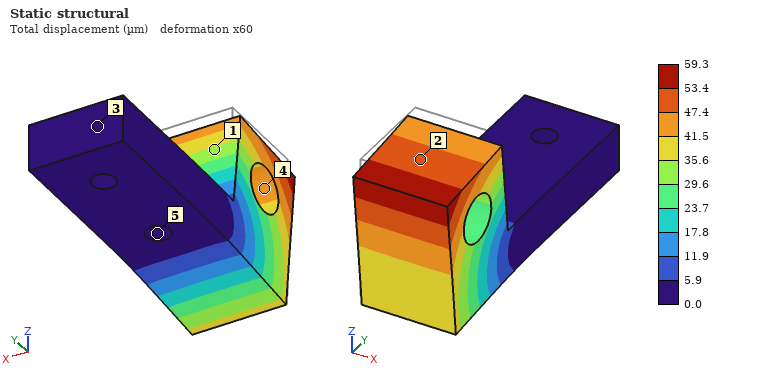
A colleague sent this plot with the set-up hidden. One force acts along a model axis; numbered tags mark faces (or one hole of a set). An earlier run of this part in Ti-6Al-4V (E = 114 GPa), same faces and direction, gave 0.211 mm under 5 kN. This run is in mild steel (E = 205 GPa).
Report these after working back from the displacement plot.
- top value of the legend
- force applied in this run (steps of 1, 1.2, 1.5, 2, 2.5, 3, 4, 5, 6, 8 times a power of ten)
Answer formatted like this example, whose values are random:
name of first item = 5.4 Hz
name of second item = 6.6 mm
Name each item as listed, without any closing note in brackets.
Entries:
top value of the legend = 59.3 µm
force applied in this run = 2.5 kN
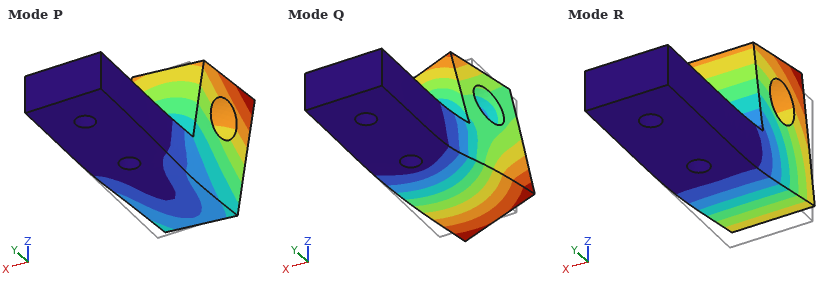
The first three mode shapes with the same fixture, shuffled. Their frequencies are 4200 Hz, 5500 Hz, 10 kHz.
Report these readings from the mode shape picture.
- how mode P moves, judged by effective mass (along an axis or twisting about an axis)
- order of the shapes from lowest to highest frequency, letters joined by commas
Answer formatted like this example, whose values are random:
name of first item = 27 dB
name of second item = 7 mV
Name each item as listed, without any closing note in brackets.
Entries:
how mode P moves, judged by effective mass = along X
order of the shapes from lowest to highest frequency, letters joined by commas = R, P, Q
